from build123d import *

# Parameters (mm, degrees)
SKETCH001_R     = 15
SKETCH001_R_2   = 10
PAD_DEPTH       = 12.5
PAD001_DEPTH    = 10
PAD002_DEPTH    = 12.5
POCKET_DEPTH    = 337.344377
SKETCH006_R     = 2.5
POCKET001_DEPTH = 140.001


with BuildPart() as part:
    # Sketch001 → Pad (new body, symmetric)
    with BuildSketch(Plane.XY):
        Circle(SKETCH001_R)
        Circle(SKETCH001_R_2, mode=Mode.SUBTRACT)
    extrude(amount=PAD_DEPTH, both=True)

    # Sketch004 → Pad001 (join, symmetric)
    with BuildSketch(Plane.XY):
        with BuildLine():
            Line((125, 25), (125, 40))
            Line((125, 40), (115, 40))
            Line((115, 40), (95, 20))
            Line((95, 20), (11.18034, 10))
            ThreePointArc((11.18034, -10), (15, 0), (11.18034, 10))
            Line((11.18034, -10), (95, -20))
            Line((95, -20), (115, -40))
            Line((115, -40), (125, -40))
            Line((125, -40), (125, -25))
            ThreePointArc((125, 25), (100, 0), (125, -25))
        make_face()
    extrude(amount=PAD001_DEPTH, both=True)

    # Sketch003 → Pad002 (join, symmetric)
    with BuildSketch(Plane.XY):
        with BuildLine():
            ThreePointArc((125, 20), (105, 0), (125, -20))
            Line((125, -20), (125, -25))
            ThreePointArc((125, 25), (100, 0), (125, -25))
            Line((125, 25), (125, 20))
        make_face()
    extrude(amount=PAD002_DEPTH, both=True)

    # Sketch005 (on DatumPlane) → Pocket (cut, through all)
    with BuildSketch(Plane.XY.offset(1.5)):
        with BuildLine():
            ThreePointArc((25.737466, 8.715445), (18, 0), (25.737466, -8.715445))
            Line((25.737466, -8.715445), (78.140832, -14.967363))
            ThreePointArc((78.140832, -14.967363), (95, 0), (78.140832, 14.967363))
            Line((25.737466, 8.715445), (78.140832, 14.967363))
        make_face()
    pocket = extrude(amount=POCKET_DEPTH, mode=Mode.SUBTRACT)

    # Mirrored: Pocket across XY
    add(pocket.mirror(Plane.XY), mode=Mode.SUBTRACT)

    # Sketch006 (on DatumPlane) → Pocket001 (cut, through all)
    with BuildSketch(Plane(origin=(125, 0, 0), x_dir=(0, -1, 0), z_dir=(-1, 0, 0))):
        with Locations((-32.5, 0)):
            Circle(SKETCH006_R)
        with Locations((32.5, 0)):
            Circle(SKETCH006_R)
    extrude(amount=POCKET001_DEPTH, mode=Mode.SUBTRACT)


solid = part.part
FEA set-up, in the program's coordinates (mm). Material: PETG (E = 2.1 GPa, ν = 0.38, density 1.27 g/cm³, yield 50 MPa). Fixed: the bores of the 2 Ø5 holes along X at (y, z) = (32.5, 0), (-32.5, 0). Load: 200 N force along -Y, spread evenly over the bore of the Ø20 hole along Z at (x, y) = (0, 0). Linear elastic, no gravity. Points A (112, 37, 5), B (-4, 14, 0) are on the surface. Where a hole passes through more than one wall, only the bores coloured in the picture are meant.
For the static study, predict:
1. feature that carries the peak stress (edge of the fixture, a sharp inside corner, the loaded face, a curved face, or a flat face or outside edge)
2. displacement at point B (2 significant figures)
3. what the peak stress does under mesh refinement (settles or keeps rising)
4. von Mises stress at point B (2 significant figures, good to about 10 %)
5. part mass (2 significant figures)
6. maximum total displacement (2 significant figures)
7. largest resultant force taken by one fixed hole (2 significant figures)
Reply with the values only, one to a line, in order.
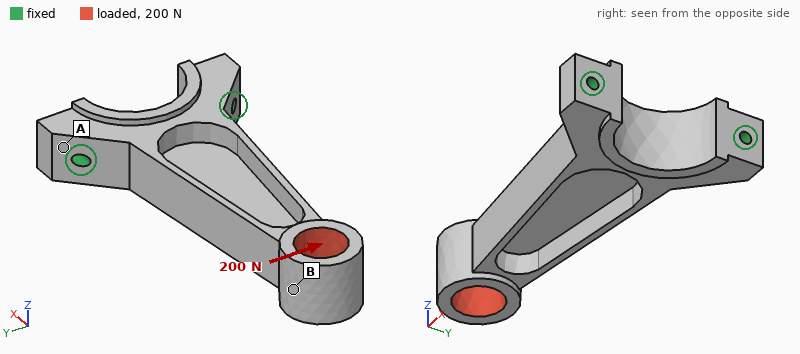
edge of the fixture
1.3 mm
keeps rising
1.6 MPa
73 g
1.5 mm
450 N
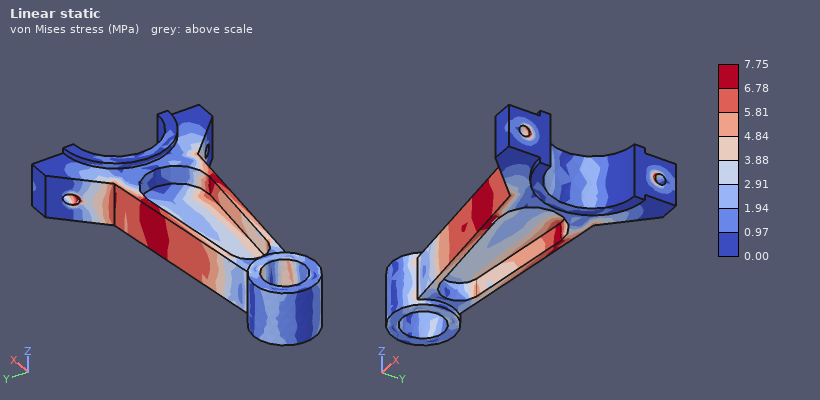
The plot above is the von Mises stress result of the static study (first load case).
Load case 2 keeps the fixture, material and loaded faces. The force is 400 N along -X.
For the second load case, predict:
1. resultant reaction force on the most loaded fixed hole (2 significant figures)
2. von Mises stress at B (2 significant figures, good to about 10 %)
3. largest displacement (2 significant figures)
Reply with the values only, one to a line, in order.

240 N
1.1 MPa
0.14 mm
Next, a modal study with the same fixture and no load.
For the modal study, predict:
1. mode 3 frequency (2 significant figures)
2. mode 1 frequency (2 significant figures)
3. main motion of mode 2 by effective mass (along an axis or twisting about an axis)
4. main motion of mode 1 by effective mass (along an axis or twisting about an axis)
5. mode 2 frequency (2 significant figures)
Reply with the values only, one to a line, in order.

600 Hz
200 Hz
along Y
along Z
510 Hz
